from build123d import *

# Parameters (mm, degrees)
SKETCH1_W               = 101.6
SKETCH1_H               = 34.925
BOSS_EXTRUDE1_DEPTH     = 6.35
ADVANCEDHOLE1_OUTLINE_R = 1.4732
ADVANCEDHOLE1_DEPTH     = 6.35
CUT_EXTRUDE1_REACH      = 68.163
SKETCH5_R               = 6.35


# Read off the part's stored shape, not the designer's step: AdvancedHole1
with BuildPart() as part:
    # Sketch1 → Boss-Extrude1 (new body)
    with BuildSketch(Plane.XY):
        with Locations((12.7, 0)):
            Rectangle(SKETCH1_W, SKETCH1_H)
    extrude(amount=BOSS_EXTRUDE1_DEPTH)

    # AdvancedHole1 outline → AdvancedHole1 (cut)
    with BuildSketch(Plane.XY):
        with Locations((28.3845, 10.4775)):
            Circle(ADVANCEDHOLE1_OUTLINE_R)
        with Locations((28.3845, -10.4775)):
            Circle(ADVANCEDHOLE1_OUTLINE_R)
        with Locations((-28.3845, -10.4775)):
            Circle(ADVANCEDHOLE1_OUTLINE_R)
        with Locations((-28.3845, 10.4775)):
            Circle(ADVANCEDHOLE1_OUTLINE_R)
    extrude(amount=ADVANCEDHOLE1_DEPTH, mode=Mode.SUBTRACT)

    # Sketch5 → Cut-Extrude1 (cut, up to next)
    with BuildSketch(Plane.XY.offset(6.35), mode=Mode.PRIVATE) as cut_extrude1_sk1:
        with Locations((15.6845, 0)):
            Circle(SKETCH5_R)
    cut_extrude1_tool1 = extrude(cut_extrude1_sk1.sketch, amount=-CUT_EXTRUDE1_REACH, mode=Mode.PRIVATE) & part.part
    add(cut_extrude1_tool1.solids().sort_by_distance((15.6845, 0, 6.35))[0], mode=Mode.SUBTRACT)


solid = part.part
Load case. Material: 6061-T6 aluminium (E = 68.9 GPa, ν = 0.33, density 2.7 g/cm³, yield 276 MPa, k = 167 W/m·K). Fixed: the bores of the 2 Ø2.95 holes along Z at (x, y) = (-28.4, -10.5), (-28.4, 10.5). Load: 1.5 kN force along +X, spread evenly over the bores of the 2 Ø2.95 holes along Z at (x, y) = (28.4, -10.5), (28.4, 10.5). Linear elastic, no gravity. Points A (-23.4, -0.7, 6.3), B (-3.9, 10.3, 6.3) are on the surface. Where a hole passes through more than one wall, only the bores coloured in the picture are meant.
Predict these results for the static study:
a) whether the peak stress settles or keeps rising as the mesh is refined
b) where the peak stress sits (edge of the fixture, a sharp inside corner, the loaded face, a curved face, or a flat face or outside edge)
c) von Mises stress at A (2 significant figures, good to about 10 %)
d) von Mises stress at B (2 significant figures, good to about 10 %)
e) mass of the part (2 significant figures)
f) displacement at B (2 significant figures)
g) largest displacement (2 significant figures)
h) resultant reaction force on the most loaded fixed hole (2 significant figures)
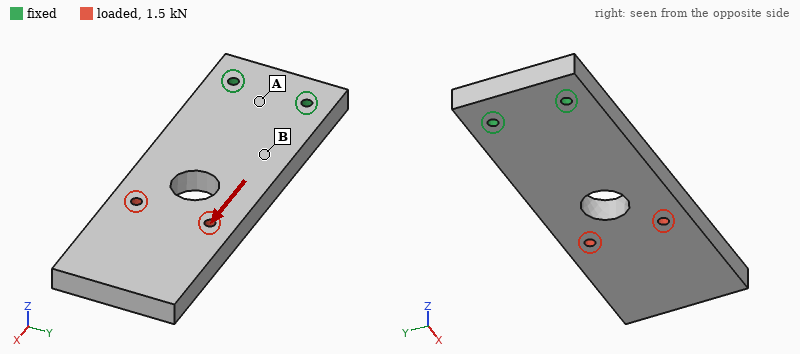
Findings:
keeps rising
edge of the fixture
3.5 MPa
7.2 MPa
58 g
2.9 µm
7.9 µm
750 N
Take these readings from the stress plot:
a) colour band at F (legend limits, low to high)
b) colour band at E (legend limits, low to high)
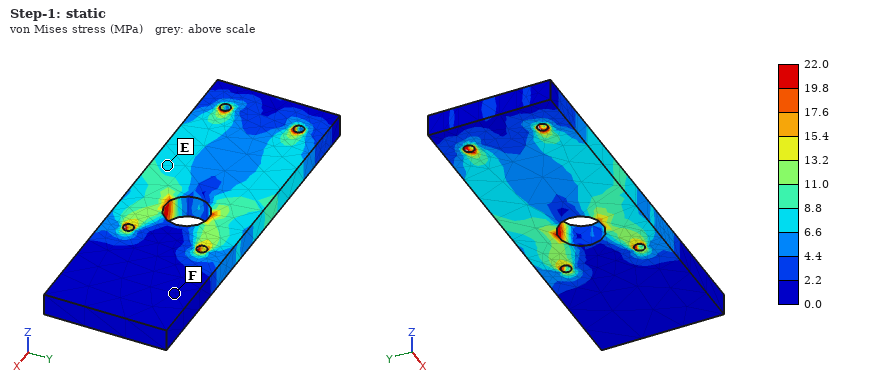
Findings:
0.0 to 2.2 MPa
6.6 to 8.8 MPa
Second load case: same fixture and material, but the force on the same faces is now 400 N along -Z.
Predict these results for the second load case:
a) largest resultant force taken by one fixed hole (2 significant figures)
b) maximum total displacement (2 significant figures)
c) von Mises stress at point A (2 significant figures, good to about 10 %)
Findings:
200 N
1.0 mm
66 MPa
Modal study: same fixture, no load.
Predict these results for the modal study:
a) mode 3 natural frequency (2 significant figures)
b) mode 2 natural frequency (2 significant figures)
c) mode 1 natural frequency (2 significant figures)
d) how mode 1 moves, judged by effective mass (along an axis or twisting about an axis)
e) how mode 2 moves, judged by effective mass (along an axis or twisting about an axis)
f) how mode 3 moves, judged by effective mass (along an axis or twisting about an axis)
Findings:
2900 Hz
2800 Hz
590 Hz
along Z
along Y
twisting about X
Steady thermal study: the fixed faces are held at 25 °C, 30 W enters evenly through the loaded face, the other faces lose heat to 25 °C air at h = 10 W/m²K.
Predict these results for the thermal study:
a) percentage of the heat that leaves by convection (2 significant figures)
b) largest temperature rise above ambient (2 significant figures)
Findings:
8.9 %
52 K
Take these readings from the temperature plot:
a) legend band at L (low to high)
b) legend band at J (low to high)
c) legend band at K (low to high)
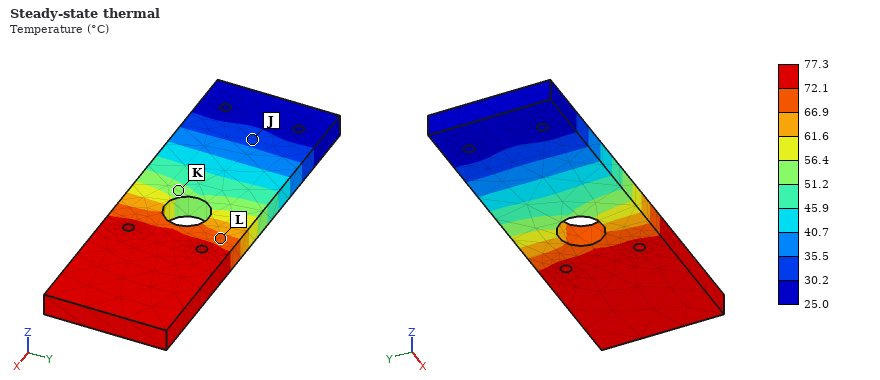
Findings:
66.9 to 72.1 °C
30.2 to 35.5 °C
51.2 to 56.4 °C
